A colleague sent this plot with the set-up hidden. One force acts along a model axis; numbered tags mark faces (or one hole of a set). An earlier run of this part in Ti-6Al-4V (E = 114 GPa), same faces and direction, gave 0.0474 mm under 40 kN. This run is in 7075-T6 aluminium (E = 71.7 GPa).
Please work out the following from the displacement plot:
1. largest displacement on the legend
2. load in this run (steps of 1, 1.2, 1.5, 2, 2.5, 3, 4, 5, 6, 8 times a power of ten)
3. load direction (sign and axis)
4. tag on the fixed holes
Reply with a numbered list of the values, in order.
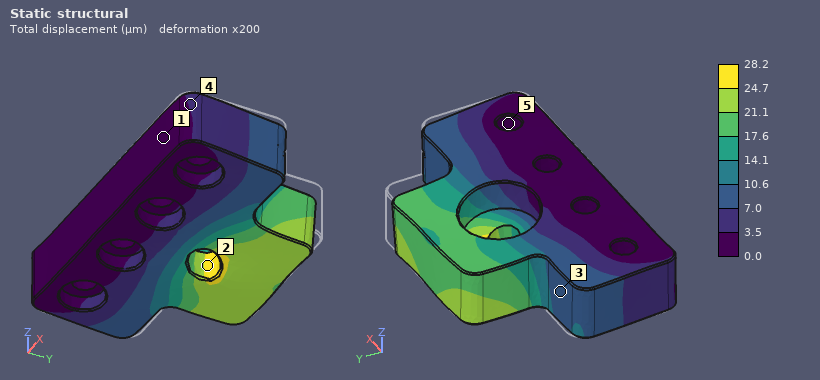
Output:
1. 28.2 µm
2. 15 kN
3. -X
4. 5
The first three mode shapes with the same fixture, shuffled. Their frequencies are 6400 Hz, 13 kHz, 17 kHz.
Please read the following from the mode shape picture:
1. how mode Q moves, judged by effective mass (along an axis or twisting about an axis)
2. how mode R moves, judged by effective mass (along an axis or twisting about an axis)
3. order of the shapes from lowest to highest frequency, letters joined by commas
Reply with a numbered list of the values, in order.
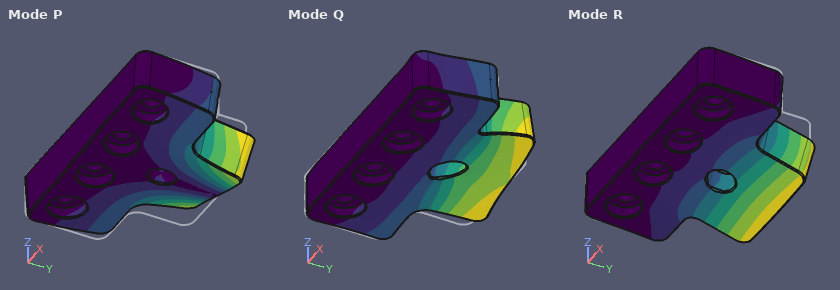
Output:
1. along X
2. along Z
3. R, P, Q
